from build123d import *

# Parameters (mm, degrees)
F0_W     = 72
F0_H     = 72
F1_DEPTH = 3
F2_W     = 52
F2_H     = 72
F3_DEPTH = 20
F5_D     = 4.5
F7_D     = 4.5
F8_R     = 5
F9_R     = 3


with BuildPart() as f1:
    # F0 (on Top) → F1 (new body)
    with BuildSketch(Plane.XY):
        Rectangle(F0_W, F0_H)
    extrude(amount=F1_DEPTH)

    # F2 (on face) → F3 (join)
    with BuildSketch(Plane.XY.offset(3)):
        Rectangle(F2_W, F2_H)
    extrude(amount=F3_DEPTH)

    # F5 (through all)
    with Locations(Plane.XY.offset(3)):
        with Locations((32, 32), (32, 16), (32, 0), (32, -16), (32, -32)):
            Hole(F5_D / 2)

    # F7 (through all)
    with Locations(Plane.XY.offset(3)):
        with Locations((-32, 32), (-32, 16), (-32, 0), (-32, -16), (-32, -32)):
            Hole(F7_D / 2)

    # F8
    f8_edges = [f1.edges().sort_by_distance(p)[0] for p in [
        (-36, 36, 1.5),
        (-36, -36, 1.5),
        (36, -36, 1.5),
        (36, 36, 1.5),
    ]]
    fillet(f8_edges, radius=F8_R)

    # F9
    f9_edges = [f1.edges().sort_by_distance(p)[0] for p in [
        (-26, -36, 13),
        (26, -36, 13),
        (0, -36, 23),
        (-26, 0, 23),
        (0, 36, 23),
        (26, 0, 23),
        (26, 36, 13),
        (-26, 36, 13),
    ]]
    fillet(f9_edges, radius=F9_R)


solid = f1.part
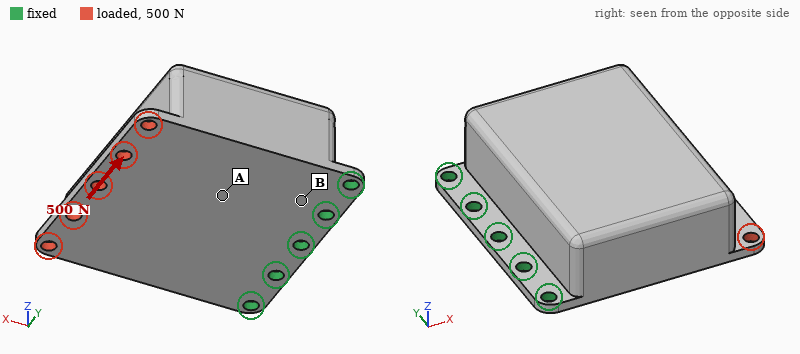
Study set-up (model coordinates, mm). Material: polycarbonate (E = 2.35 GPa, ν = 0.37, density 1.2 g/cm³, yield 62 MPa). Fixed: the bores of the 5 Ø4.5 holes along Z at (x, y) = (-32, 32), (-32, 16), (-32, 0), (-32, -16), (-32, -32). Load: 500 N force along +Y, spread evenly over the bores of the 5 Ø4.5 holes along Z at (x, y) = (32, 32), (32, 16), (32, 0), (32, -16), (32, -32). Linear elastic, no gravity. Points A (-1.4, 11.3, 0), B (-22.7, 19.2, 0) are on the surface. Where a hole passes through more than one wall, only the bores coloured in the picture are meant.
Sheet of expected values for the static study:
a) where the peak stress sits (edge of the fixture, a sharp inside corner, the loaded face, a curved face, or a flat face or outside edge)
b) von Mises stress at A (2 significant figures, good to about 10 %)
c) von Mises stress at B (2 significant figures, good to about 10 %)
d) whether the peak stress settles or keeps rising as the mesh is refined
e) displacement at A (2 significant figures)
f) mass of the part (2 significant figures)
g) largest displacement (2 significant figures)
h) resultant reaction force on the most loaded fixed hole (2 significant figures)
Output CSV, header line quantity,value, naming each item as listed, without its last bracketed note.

quantity,value
where the peak stress sits,edge of the fixture
von Mises stress at A,2.5 MPa
von Mises stress at B,4.8 MPa
whether the peak stress settles or keeps rising as the mesh is refined,keeps rising
displacement at A,0.11 mm
mass of the part,110 g
largest displacement,0.32 mm
resultant reaction force on the most loaded fixed hole,400 N
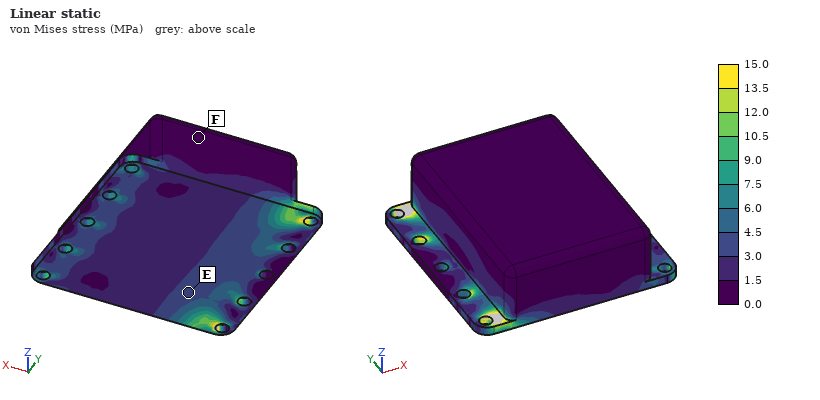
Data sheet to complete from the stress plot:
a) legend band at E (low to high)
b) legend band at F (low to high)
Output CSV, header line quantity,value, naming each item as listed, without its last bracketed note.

quantity,value
legend band at E,3.0 to 4.5 MPa
legend band at F,0.0 to 1.5 MPa
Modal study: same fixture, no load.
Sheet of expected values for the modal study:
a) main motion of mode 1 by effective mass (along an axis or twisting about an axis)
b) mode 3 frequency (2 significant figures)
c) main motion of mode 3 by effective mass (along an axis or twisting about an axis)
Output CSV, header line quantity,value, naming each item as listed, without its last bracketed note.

quantity,value
main motion of mode 1 by effective mass,along Z
mode 3 frequency,1300 Hz
main motion of mode 3 by effective mass,along Y
